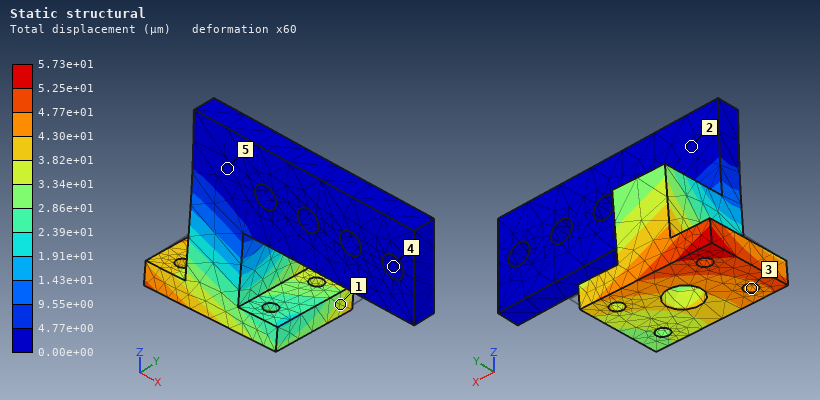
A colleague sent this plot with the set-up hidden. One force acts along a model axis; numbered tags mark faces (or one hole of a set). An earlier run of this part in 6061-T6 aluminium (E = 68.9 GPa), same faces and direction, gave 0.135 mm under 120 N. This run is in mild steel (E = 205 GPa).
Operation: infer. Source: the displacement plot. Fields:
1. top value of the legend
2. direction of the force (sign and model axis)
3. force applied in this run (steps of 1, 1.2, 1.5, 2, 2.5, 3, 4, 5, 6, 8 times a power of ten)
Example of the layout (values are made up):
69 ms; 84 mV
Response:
5.73e+01 µm; -Y; 150 N
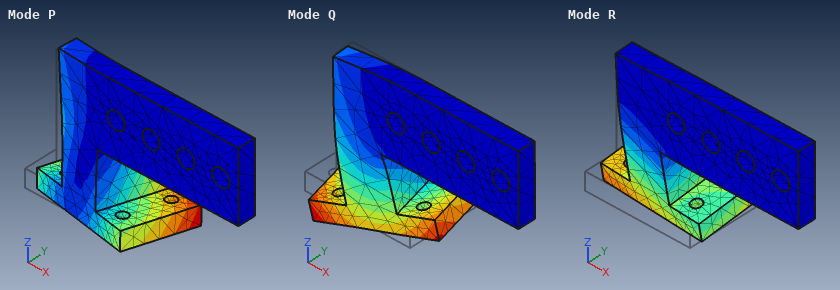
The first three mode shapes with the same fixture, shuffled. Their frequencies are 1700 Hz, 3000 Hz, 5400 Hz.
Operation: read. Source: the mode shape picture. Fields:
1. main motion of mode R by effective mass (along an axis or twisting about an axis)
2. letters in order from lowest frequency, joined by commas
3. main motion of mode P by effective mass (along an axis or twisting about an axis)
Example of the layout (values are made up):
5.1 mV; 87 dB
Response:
along Y; R, P, Q; along X
